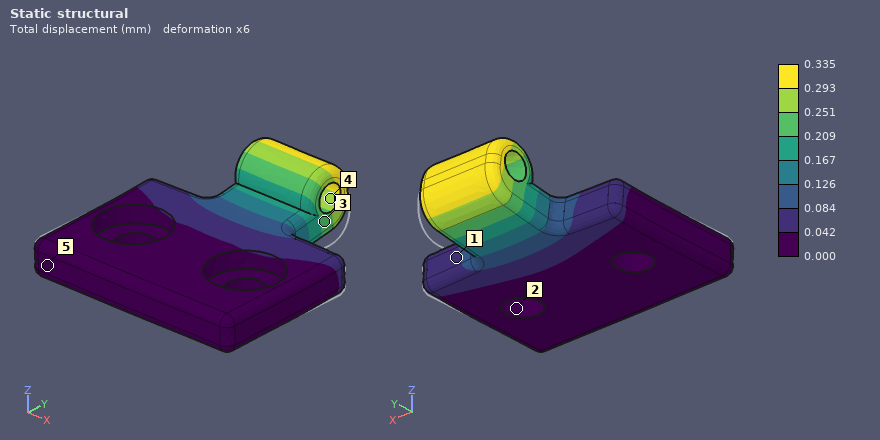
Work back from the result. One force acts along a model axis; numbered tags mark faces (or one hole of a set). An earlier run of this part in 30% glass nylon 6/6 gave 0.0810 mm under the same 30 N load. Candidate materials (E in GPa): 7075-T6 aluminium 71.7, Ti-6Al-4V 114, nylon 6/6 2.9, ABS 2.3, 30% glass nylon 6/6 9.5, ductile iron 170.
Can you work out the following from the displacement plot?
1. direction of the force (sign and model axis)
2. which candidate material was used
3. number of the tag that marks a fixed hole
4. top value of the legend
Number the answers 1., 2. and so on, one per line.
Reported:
1. +Z
2. ABS
3. 2
4. 0.335 mm
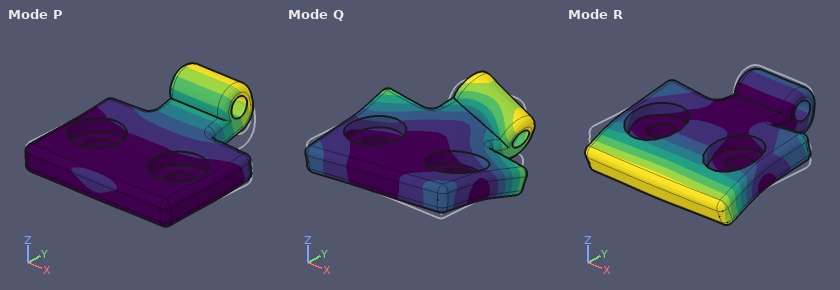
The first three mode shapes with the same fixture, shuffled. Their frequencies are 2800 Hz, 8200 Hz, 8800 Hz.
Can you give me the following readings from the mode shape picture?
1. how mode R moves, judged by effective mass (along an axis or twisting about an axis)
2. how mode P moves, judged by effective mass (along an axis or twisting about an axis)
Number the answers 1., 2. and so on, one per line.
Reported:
1. along Z
2. along Z
